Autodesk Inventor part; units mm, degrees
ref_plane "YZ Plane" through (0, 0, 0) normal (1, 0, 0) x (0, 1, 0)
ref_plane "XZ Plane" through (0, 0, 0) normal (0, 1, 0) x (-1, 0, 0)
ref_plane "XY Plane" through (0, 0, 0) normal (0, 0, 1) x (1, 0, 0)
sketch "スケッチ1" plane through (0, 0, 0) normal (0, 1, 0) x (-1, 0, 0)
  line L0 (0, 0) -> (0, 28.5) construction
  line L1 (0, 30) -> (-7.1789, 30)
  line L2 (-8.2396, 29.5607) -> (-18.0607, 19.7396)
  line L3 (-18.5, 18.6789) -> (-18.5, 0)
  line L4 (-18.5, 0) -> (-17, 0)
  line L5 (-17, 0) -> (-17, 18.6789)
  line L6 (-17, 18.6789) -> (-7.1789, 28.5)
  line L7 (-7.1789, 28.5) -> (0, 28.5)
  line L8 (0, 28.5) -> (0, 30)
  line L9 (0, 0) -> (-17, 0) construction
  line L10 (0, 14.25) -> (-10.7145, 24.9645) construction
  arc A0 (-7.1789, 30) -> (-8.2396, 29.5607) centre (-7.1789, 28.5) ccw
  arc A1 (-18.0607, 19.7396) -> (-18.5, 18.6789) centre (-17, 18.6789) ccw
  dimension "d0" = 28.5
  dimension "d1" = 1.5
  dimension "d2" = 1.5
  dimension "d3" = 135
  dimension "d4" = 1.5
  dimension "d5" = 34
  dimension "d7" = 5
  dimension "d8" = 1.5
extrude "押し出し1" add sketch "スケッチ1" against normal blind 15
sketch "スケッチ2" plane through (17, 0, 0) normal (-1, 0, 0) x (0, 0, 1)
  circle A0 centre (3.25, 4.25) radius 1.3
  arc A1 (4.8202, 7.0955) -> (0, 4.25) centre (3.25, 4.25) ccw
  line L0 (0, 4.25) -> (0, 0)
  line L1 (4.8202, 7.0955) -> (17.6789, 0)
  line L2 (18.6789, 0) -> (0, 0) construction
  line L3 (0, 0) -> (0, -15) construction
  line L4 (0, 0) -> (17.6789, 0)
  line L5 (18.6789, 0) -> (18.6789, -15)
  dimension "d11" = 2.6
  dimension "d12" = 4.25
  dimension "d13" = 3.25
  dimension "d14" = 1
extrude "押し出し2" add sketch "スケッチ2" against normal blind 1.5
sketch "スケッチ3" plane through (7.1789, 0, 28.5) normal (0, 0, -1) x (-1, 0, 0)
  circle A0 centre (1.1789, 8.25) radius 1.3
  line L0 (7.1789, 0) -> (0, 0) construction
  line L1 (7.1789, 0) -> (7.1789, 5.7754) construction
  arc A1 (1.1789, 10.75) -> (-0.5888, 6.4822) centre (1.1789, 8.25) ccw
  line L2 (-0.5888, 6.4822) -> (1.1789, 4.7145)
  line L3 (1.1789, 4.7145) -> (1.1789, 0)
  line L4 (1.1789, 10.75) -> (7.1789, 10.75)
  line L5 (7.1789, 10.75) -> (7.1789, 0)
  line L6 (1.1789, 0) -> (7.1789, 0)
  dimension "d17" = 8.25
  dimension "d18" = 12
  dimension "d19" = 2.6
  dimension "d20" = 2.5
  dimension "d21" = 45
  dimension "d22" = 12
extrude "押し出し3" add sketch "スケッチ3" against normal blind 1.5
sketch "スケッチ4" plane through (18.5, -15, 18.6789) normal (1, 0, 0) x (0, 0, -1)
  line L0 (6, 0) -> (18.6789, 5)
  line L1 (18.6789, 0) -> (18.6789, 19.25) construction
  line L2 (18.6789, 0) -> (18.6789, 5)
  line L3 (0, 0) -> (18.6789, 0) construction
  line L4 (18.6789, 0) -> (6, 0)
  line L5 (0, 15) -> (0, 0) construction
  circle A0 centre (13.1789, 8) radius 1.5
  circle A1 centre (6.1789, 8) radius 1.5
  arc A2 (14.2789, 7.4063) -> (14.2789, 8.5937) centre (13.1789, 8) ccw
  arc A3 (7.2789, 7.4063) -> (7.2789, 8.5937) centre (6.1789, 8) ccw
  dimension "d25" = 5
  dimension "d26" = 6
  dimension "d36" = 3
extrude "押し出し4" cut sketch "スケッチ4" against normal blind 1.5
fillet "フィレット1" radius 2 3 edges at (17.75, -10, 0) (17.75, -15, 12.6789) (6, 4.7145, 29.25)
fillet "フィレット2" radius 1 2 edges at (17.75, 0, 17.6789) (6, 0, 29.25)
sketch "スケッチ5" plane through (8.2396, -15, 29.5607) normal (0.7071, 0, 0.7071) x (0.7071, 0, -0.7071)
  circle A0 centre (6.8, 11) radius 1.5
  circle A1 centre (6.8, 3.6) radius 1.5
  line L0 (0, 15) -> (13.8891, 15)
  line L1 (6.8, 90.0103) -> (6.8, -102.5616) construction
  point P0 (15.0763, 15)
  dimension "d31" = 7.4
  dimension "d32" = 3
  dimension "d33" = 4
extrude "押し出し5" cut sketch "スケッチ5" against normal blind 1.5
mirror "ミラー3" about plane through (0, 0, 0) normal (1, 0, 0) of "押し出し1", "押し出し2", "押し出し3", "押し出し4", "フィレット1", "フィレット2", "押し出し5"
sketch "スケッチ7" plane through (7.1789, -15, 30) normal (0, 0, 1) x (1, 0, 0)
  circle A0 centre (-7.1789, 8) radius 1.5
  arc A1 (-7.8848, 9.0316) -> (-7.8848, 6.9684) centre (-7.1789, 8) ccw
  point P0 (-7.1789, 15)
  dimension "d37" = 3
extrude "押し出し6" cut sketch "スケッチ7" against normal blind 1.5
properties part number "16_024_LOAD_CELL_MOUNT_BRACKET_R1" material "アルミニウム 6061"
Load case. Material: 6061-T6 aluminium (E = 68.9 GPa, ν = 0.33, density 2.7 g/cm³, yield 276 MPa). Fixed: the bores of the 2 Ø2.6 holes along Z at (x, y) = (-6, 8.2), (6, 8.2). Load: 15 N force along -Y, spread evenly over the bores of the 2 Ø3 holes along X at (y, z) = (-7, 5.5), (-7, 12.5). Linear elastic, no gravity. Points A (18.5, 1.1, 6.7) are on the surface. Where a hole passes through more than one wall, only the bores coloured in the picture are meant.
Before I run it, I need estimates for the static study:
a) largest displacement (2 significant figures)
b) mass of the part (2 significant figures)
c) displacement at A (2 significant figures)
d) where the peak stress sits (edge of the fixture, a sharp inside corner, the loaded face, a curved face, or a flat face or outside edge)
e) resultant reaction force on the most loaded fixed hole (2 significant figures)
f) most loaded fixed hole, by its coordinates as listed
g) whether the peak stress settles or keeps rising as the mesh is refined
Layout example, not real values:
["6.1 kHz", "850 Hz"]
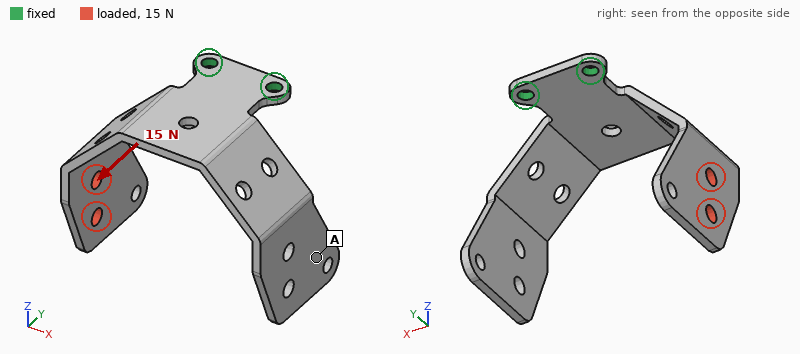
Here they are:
["0.59 mm", "5.6 g", "0.28 mm", "a sharp inside corner", "31 N", "(-6, 8.2)", "keeps rising"]
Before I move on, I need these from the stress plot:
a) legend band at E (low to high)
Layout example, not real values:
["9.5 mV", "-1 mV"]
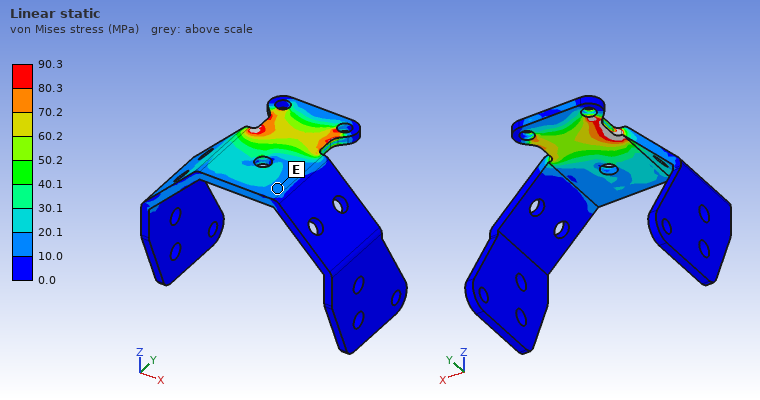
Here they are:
["10.0 to 20.1 MPa"]
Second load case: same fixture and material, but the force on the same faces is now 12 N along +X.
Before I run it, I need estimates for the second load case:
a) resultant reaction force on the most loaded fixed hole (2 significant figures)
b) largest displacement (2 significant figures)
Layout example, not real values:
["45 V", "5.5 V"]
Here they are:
["28 N", "0.60 mm"]
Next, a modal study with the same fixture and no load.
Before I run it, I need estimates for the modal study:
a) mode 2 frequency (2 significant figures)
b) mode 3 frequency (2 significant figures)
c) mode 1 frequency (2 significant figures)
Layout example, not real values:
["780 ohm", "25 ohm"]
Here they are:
["570 Hz", "790 Hz", "570 Hz"]
